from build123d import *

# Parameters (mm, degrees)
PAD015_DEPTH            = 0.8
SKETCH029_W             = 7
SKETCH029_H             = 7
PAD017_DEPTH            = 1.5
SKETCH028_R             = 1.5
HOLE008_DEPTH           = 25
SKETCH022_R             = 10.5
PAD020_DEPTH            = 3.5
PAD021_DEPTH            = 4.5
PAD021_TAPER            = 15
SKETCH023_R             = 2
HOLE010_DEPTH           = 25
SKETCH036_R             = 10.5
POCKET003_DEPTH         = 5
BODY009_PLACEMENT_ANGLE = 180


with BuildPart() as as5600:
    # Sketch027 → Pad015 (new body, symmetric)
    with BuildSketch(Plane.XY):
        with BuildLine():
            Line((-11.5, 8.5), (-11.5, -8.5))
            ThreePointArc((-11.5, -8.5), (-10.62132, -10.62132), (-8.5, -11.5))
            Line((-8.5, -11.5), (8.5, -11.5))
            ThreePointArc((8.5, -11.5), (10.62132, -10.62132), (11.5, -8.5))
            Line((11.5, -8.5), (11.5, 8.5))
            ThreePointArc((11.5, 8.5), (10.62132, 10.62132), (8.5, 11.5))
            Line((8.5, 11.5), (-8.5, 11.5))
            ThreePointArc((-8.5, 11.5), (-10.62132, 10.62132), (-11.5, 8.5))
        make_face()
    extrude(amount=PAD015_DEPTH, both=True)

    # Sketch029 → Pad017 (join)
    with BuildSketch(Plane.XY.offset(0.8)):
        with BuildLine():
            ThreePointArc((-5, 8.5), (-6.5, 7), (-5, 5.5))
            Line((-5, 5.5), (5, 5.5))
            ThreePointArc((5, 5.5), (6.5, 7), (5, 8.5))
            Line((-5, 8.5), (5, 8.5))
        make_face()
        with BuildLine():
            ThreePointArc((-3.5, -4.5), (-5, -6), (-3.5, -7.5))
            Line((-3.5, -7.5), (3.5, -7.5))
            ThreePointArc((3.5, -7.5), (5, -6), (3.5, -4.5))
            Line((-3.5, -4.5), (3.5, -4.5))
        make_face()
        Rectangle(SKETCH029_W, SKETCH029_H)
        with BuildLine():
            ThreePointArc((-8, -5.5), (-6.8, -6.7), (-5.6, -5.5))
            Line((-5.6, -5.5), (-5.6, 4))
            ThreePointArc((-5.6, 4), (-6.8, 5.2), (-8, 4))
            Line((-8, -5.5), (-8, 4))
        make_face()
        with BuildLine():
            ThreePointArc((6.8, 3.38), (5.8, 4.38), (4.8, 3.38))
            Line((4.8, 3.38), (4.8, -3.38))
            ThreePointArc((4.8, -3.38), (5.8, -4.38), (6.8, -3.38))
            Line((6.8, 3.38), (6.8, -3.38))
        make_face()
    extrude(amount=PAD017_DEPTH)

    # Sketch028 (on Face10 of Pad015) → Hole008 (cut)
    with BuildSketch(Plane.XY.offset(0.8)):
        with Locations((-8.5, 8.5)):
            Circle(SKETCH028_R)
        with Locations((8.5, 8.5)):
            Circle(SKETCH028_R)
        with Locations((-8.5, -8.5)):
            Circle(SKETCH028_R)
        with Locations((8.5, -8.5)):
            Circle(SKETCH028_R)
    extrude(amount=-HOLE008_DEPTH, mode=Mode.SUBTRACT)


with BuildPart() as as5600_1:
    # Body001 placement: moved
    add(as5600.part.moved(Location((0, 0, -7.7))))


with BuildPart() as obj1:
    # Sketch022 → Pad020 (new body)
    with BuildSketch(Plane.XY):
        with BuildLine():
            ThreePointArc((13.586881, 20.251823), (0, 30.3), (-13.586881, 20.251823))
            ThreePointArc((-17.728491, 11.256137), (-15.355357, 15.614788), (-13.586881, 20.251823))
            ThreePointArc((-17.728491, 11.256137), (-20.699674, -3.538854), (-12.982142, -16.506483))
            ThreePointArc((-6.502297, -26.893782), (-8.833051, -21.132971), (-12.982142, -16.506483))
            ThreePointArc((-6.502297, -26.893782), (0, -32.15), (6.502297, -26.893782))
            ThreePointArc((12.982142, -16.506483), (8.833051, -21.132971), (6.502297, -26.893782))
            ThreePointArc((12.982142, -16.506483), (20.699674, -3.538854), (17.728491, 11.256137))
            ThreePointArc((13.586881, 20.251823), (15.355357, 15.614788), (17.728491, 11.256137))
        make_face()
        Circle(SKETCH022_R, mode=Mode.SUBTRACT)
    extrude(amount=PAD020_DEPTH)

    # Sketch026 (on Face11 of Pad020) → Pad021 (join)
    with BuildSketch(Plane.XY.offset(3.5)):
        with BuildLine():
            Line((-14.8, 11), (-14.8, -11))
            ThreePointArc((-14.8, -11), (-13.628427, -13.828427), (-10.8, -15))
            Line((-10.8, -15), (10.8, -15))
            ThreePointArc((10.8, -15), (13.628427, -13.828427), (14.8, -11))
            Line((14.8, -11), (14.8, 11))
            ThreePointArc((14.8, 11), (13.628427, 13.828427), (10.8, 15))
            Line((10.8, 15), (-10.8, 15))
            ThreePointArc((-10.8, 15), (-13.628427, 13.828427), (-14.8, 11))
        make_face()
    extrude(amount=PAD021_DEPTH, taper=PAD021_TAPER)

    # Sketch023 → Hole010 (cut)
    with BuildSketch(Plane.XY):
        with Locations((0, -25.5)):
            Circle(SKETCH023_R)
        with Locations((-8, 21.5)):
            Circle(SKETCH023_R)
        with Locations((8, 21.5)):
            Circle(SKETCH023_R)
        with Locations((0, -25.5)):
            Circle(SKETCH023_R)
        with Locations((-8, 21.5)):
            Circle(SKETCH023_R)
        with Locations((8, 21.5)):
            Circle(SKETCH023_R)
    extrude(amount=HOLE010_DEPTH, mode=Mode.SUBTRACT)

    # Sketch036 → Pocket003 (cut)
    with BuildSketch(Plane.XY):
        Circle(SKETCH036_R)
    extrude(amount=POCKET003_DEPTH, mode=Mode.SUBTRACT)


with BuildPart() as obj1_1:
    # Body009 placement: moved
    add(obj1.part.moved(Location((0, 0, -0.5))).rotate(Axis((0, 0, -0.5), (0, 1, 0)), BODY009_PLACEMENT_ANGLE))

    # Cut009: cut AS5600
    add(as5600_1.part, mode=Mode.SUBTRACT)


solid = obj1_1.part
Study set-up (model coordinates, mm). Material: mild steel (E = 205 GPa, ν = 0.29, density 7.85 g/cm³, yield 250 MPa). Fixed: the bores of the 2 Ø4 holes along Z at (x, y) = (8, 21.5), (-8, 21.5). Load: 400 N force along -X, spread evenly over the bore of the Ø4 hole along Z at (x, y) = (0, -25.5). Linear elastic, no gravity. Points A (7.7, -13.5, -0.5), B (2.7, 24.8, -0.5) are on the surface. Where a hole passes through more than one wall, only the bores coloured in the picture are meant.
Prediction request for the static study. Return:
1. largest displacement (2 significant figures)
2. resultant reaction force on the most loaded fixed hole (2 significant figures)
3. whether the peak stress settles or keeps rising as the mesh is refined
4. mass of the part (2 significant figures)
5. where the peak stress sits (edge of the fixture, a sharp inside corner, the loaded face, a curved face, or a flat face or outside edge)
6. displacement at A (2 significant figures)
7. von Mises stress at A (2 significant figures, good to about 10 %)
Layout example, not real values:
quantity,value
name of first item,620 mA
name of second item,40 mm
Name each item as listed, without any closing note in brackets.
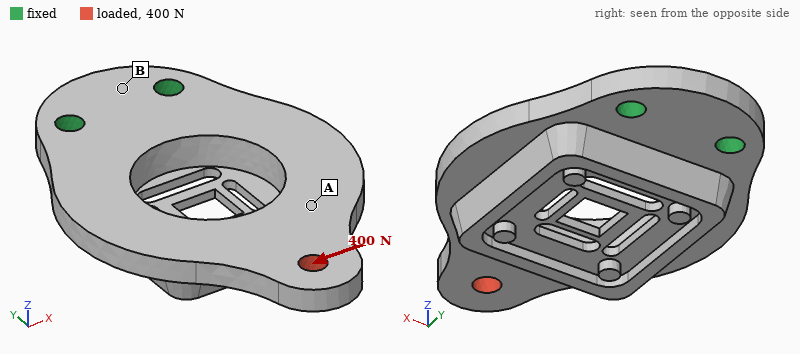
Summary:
quantity,value
largest displacement,20 µm
resultant reaction force on the most loaded fixed hole,1.0 kN
whether the peak stress settles or keeps rising as the mesh is refined,keeps rising
mass of the part,55 g
where the peak stress sits,edge of the fixture
displacement at A,15 µm
von Mises stress at A,14 MPa
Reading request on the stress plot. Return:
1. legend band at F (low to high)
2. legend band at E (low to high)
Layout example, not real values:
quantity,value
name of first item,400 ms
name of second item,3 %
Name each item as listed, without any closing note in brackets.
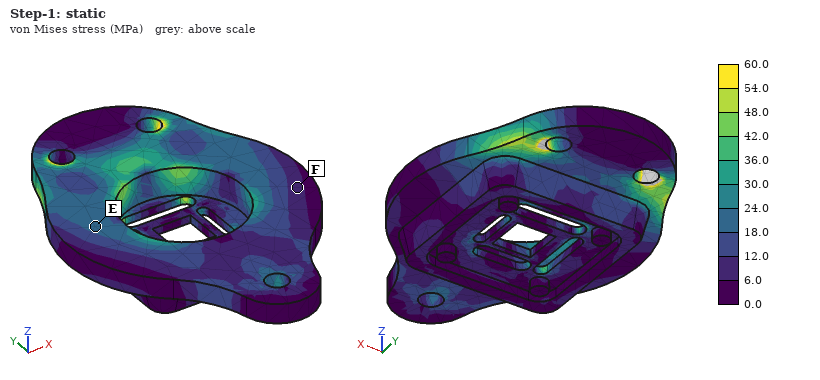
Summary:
quantity,value
legend band at F,6.0 to 12.0 MPa
legend band at E,18.0 to 24.0 MPa
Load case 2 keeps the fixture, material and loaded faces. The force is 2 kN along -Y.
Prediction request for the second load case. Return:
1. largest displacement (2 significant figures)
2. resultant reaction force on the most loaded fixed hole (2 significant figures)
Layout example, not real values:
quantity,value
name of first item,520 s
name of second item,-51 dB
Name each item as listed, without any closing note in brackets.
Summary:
quantity,value
largest displacement,45 µm
resultant reaction force on the most loaded fixed hole,1.0 kN
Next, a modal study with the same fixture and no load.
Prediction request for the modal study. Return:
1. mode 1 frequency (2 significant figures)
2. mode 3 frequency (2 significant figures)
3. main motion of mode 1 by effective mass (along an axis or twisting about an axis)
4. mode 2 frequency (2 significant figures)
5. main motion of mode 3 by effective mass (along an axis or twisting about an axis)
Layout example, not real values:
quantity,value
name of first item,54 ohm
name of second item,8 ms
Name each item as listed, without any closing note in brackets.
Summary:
quantity,value
mode 1 frequency,1500 Hz
mode 3 frequency,6200 Hz
main motion of mode 1 by effective mass,along Z
mode 2 frequency,4700 Hz
main motion of mode 3 by effective mass,along X
